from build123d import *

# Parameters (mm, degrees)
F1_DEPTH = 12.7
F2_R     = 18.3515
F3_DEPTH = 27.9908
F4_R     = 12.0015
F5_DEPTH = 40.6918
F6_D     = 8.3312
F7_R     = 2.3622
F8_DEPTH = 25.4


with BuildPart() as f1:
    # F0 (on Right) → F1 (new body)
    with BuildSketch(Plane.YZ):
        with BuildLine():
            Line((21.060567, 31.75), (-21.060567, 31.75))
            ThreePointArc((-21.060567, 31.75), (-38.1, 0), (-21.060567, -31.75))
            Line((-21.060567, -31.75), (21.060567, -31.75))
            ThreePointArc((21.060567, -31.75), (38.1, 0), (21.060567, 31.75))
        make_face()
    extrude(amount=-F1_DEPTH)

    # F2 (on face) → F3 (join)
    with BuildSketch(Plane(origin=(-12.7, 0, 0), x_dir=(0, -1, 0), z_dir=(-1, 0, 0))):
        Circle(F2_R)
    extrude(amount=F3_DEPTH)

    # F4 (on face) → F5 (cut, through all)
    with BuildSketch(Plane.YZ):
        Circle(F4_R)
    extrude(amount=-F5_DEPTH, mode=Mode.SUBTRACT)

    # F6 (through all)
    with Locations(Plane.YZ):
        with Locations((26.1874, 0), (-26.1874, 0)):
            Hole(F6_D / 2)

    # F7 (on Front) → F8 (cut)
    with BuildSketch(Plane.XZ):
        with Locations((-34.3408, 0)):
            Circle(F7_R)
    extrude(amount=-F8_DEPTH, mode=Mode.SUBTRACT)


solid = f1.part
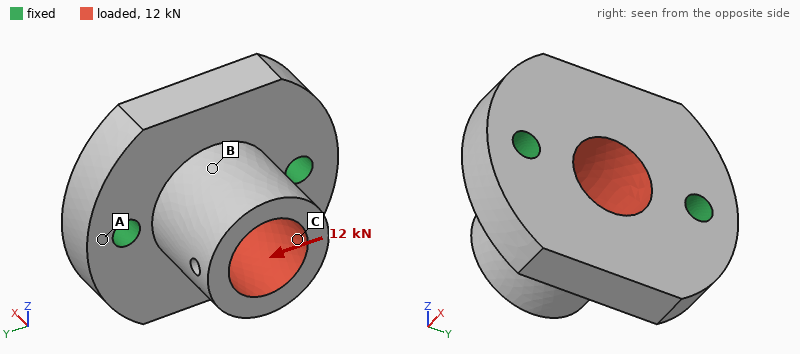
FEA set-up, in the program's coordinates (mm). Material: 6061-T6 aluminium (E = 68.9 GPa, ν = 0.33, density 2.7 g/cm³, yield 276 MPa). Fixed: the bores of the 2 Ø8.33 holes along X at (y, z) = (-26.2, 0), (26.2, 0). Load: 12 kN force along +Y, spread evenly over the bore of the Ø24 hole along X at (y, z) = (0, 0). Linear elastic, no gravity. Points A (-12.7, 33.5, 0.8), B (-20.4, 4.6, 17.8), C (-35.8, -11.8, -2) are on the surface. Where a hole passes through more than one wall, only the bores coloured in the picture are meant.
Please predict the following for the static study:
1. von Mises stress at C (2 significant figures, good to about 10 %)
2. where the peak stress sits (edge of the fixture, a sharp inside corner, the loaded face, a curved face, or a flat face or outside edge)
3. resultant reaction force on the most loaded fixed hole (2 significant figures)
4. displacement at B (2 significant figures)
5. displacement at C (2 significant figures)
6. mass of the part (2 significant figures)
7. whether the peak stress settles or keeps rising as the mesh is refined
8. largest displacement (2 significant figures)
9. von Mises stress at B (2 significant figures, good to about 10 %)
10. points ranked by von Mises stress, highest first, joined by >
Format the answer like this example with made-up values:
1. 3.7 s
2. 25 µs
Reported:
1. 11 MPa
2. a sharp inside corner
3. 7.0 kN
4. 14 µm
5. 30 µm
6. 170 g
7. keeps rising
8. 34 µm
9. 21 MPa
10. B > C > A
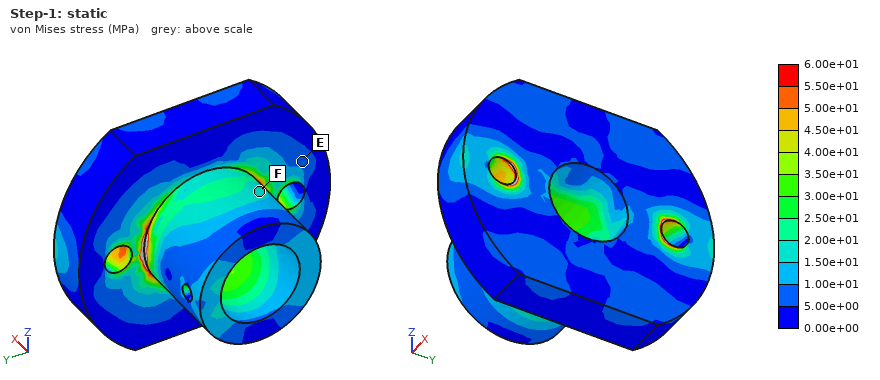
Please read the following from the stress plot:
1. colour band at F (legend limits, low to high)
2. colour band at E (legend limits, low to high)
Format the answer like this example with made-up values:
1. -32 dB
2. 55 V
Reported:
1. 1.50e+01 to 2.00e+01 MPa
2. 5.00e+00 to 1.00e+01 MPa
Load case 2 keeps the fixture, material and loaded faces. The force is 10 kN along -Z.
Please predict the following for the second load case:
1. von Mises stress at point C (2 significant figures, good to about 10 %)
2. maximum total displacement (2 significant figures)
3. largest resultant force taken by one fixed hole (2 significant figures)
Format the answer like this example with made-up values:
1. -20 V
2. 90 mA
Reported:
1. 14 MPa
2. 79 µm
3. 5.0 kN
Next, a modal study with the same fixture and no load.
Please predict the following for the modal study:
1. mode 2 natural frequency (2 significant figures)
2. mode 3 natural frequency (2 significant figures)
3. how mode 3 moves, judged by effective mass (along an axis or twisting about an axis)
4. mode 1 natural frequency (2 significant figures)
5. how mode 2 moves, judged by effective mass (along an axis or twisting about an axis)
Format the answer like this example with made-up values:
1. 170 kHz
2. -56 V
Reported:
1. 10 kHz
2. 13 kHz
3. along Y
4. 6100 Hz
5. along X
